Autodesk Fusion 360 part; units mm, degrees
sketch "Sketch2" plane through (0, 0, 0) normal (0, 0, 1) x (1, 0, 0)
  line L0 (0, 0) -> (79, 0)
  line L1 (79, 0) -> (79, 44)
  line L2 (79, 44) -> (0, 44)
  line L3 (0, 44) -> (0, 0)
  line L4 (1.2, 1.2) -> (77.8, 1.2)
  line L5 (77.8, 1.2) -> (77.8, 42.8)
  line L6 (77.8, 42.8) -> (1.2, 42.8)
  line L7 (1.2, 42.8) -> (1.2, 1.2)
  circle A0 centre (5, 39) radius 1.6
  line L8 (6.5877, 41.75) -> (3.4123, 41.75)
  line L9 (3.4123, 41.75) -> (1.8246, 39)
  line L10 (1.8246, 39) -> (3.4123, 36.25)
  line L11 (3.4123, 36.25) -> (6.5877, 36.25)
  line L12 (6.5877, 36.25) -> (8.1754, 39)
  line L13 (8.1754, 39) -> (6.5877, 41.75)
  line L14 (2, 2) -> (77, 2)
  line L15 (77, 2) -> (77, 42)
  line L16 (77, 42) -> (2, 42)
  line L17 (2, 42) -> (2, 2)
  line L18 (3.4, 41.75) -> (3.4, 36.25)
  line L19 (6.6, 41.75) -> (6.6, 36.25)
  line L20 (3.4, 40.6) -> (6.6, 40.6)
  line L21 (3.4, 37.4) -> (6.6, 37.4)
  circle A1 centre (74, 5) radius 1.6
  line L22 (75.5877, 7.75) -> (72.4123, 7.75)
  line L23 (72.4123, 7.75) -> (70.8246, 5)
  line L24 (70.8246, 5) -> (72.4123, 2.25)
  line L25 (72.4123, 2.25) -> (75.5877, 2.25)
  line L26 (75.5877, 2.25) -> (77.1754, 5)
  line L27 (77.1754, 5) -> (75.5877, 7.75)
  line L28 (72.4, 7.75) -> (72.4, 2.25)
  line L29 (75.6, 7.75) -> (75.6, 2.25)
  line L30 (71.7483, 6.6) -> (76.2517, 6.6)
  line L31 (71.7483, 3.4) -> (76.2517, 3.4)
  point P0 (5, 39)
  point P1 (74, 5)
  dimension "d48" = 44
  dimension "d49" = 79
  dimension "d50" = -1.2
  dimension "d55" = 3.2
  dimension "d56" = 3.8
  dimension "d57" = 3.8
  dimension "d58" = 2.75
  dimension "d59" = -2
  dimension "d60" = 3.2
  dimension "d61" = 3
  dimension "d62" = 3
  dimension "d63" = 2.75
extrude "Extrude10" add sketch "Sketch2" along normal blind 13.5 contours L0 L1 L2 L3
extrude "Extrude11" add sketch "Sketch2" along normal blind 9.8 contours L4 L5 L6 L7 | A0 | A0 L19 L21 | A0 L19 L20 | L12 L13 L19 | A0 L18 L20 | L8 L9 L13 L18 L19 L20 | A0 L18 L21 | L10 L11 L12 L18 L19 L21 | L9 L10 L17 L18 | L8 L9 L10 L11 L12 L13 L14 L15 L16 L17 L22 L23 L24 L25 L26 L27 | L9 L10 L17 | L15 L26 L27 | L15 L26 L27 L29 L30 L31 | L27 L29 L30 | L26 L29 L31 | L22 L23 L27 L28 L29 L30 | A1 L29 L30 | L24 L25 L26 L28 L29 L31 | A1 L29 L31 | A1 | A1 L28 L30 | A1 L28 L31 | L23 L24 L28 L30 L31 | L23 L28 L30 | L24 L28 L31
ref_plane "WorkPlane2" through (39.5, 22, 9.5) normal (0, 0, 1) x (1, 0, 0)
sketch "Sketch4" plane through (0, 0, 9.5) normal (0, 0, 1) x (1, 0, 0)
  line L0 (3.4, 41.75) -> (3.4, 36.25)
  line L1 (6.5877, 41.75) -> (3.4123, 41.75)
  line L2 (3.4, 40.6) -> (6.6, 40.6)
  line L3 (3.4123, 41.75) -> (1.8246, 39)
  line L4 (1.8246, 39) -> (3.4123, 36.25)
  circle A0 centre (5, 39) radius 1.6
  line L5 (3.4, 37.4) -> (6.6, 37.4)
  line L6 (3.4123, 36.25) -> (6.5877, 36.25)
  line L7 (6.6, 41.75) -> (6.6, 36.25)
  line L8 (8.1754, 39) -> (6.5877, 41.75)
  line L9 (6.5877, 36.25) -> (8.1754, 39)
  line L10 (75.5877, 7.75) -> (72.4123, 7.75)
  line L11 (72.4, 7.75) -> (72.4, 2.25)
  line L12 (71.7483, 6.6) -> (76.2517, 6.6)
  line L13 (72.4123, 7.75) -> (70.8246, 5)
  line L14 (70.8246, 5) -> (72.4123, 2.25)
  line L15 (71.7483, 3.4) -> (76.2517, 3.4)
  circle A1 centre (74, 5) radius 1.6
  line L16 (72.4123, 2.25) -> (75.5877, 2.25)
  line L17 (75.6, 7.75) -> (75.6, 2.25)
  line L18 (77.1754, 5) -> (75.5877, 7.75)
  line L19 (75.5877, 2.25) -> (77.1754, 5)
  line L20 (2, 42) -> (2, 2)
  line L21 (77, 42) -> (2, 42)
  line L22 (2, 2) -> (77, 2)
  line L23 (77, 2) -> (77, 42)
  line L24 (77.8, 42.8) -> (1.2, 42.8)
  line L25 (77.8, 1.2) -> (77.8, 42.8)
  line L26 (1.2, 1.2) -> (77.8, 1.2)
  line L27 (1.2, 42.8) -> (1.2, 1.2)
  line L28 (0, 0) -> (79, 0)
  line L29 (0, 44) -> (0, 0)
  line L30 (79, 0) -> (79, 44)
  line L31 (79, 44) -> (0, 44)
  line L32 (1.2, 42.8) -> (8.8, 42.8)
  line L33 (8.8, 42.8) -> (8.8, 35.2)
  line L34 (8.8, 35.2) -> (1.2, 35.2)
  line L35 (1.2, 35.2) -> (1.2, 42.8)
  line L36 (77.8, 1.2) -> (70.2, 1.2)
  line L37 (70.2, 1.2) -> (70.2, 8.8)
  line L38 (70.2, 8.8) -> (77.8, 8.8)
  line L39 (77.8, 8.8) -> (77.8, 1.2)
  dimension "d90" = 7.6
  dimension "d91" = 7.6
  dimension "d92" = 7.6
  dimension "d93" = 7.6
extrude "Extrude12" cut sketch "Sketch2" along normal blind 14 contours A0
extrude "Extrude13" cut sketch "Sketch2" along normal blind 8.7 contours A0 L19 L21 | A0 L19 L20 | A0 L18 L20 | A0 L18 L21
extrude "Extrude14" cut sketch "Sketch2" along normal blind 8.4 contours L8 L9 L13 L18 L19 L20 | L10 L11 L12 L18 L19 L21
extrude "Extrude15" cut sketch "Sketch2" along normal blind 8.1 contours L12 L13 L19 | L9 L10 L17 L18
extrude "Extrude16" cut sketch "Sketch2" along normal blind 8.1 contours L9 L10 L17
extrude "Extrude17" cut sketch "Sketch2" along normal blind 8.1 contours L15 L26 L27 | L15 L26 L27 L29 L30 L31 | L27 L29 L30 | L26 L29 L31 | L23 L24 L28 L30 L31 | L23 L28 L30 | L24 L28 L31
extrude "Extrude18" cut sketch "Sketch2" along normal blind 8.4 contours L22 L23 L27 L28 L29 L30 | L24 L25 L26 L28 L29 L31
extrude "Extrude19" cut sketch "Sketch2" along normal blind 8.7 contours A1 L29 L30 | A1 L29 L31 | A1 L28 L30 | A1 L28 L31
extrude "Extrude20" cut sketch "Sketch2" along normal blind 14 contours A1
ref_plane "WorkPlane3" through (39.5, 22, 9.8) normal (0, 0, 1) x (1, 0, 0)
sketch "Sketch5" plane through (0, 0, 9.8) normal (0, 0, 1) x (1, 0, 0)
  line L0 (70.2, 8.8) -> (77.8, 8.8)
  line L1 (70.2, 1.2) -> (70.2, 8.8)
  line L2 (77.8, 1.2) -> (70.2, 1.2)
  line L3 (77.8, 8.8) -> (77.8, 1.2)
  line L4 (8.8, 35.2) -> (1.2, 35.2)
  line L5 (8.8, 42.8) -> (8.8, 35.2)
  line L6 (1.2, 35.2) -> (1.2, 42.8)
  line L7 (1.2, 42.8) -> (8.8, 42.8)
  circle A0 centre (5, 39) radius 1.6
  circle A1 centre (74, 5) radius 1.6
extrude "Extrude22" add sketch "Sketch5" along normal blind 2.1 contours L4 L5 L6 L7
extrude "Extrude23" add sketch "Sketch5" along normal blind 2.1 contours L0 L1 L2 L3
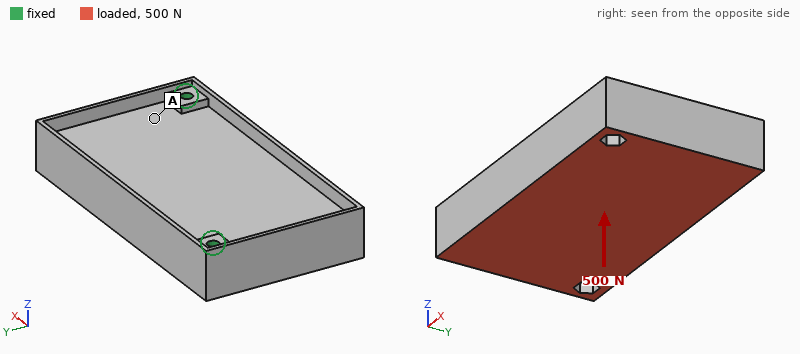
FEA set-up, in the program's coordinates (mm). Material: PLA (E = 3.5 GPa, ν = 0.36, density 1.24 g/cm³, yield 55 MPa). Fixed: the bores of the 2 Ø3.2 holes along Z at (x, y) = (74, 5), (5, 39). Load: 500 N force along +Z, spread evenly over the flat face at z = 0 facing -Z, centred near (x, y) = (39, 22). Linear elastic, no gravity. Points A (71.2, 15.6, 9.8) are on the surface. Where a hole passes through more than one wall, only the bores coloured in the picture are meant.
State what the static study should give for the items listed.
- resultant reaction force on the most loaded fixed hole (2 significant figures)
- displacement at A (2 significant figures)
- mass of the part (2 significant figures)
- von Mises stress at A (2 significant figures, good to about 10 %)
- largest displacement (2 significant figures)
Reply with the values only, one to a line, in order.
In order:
400 N
0.074 mm
43 g
1.7 MPa
0.22 mm
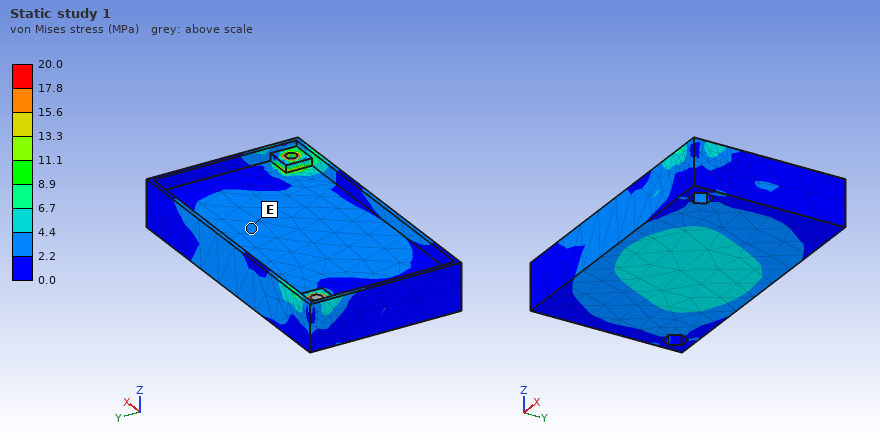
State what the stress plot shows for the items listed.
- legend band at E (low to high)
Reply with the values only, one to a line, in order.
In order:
2.2 to 4.4 MPa
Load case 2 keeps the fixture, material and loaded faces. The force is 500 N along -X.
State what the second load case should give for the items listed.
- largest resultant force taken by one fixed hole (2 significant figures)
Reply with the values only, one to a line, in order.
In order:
260 N
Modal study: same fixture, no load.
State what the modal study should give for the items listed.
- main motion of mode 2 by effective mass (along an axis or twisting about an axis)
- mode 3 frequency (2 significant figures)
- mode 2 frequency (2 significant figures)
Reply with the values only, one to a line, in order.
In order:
along Z
2700 Hz
1400 Hz
